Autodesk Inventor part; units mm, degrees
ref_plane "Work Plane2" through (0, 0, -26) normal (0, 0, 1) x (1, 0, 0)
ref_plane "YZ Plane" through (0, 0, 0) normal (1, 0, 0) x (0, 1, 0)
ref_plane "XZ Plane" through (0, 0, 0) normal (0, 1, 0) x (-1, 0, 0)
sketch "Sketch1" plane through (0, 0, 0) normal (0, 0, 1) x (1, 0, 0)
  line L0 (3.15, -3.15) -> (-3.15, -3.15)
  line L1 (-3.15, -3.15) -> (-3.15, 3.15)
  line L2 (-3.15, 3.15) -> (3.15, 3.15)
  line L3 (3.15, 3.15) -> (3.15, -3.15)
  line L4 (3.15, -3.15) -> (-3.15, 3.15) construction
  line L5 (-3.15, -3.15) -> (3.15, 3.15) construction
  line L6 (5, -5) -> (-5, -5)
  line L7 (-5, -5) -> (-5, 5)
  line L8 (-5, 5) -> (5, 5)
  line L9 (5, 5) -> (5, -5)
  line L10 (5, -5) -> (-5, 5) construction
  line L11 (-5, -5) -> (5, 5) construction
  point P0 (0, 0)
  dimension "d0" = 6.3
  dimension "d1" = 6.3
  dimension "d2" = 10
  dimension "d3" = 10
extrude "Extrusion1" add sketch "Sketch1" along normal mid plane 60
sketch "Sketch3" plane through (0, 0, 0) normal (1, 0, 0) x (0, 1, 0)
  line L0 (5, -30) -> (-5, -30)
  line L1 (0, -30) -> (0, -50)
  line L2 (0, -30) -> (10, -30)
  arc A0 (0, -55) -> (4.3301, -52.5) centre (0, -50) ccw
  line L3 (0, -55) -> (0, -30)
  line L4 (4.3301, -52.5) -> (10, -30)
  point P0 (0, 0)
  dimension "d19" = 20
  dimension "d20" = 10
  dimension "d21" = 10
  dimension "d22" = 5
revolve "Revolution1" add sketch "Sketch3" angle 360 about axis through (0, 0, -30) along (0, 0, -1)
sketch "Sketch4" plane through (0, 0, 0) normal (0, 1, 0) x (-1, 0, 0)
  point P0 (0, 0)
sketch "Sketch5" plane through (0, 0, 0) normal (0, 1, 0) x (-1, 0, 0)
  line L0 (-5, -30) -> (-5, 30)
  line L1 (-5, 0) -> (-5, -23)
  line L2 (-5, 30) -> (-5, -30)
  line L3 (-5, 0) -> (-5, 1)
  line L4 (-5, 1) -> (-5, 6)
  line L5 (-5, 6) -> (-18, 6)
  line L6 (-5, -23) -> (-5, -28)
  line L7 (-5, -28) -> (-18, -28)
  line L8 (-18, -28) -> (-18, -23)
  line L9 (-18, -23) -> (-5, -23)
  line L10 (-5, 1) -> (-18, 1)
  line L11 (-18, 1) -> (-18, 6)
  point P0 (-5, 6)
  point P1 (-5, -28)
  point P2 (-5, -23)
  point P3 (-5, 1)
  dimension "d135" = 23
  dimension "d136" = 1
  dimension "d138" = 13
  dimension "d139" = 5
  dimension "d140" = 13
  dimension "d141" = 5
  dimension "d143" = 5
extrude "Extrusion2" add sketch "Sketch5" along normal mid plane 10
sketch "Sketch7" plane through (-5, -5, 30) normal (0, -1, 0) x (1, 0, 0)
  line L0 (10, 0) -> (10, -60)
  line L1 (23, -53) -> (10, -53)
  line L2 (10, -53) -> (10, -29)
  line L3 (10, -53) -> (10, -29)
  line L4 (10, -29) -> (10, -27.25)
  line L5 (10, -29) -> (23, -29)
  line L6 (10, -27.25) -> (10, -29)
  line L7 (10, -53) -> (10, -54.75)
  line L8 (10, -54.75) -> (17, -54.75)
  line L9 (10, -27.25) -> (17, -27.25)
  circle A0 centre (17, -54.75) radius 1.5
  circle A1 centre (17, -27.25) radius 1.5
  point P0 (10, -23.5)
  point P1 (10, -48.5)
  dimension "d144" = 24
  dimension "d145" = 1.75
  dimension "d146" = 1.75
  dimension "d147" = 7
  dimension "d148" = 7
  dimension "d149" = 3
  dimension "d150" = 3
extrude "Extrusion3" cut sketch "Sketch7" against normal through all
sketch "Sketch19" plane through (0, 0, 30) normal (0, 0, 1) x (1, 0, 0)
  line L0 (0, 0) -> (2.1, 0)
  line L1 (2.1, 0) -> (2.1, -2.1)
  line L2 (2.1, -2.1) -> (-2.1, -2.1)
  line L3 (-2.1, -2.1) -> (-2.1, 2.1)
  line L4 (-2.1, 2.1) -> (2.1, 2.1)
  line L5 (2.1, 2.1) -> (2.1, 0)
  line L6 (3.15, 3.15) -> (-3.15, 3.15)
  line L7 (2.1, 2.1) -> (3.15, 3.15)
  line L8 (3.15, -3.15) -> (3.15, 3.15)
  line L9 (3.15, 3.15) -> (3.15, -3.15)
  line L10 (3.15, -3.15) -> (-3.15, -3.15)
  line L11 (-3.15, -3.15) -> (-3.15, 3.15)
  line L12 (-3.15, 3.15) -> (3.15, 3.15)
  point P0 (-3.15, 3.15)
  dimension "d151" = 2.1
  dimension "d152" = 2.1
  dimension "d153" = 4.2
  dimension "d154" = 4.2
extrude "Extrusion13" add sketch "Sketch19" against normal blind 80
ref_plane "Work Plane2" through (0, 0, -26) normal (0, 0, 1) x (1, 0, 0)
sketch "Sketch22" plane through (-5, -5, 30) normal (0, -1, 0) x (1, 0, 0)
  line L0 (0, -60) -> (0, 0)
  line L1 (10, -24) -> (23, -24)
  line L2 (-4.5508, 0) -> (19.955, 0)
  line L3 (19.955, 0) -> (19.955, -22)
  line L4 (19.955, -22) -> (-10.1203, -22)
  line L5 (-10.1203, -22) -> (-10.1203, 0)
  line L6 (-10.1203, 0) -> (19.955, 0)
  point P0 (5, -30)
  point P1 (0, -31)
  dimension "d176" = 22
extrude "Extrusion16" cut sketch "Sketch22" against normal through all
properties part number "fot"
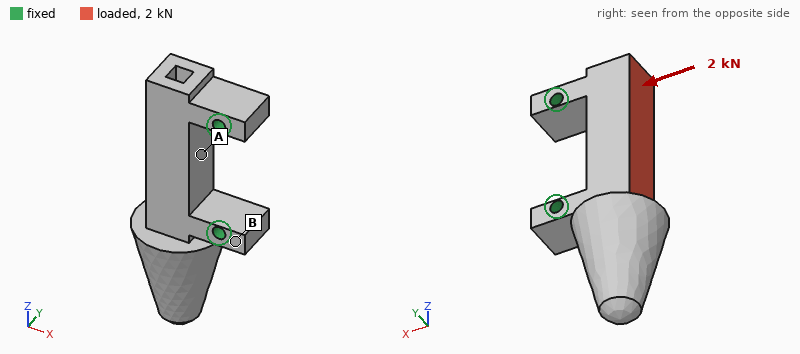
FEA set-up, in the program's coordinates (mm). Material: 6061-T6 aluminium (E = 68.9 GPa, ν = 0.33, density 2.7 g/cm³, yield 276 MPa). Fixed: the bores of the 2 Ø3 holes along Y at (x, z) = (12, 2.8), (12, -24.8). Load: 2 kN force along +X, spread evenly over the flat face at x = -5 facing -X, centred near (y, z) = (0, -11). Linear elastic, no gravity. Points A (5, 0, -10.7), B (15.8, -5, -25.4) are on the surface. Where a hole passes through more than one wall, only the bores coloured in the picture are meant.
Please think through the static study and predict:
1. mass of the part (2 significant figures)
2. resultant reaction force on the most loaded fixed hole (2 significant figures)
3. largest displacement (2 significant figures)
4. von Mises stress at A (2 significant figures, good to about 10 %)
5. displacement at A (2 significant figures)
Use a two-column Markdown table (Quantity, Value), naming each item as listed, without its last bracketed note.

| Quantity | Value |
|---|---|
| mass of the part | 22 g |
| resultant reaction force on the most loaded fixed hole | 1.0 kN |
| largest displacement | 10 µm |
| von Mises stress at A | 18 MPa |
| displacement at A | 9.1 µm |
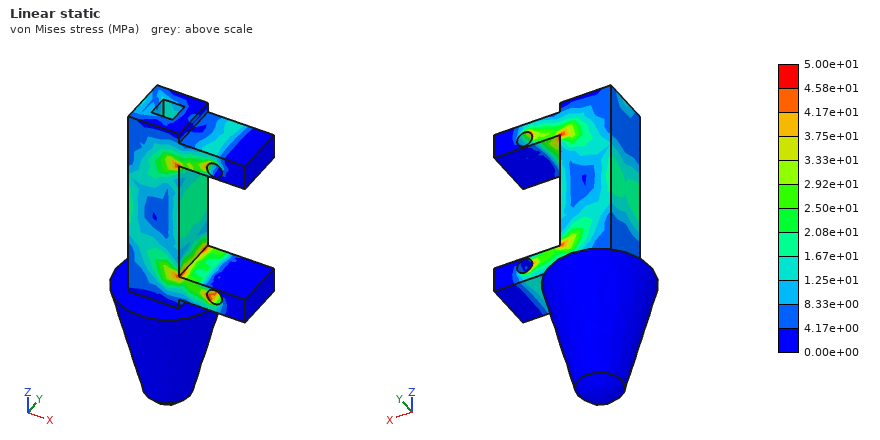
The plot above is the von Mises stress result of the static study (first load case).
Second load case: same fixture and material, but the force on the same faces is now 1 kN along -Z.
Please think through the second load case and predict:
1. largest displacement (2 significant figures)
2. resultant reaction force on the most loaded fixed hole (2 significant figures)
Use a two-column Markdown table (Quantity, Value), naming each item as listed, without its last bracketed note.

| Quantity | Value |
|---|---|
| largest displacement | 23 µm |
| resultant reaction force on the most loaded fixed hole | 650 N |
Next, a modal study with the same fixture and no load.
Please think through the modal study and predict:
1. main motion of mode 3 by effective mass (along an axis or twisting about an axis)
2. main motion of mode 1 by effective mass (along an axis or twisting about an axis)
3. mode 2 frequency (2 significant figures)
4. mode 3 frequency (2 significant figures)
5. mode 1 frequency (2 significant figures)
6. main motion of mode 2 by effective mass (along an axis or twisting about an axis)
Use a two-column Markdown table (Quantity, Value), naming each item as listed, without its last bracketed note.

| Quantity | Value |
|---|---|
| main motion of mode 3 by effective mass | along Y |
| main motion of mode 1 by effective mass | along Y |
| mode 2 frequency | 6700 Hz |
| mode 3 frequency | 11 kHz |
| mode 1 frequency | 5200 Hz |
| main motion of mode 2 by effective mass | along X |
